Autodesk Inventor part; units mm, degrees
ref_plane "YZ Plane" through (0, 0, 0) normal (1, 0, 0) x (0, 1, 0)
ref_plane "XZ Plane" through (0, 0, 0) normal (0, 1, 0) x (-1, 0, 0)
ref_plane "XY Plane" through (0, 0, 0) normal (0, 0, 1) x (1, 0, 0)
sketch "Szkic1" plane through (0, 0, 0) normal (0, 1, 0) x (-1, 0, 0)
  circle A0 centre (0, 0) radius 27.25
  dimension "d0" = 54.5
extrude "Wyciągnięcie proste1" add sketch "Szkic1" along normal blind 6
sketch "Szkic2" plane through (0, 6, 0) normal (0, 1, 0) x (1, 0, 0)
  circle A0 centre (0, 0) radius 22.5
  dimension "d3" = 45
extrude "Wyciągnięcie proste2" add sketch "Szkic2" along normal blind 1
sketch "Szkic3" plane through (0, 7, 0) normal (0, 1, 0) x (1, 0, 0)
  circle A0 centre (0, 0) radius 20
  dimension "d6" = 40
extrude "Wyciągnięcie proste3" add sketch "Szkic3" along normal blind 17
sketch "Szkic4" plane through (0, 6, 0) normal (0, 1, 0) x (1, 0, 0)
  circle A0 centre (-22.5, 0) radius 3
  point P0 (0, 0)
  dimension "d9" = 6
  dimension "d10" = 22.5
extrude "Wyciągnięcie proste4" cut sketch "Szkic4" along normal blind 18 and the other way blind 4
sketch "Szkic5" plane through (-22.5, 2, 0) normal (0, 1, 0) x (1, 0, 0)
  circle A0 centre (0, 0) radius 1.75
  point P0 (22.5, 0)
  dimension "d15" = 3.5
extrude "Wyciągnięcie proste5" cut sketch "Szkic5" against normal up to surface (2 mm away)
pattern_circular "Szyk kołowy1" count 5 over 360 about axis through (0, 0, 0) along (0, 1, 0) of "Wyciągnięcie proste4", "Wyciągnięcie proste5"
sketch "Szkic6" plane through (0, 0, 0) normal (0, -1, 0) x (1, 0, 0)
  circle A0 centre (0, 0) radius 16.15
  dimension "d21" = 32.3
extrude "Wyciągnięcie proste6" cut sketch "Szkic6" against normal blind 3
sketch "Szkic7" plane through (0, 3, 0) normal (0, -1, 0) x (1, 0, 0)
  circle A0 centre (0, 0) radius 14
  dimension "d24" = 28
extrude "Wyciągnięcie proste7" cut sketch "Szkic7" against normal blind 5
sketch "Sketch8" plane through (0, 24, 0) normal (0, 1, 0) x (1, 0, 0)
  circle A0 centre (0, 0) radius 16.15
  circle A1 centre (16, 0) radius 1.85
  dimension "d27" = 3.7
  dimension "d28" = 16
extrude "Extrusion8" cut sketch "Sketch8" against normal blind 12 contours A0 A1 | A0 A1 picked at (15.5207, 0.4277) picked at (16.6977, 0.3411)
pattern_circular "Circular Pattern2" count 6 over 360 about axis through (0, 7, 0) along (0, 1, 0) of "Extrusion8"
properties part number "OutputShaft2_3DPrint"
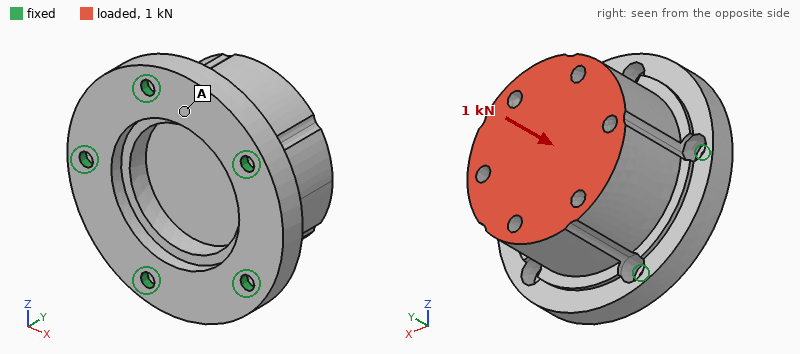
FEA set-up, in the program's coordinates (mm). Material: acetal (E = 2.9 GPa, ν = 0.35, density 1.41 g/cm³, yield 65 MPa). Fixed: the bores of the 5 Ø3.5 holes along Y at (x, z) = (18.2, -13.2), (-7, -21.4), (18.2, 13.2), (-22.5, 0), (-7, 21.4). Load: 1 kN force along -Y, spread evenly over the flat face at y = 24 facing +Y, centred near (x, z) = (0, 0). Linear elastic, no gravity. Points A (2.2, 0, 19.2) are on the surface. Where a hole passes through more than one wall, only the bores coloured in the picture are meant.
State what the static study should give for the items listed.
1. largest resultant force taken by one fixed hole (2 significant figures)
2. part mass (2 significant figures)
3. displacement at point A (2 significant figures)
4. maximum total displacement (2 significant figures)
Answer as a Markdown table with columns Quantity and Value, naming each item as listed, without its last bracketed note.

| Quantity | Value |
|---|---|
| largest resultant force taken by one fixed hole | 230 N |
| part mass | 42 g |
| displacement at point A | 31 µm |
| maximum total displacement | 41 µm |
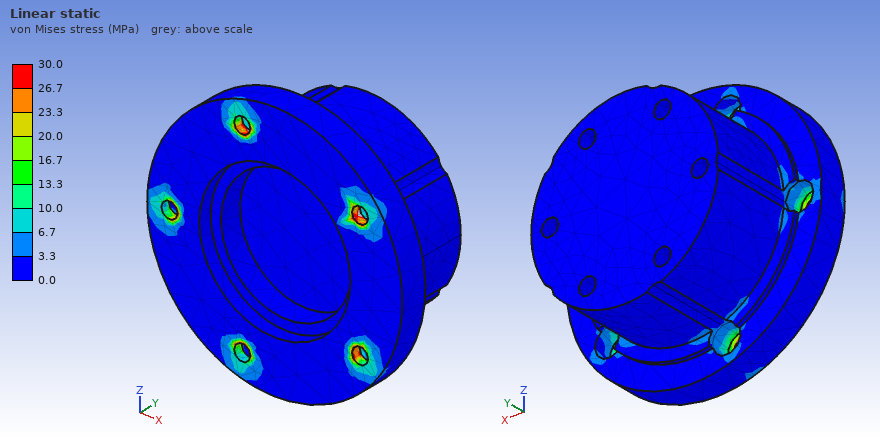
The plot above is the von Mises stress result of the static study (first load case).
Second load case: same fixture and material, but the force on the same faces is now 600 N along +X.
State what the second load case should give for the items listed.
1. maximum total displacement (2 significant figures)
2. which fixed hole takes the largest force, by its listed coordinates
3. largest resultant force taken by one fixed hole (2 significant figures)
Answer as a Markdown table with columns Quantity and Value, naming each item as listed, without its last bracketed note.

| Quantity | Value |
|---|---|
| maximum total displacement | 75 µm |
| which fixed hole takes the largest force, by its listed coordinates | (-22.5, 0) |
| largest resultant force taken by one fixed hole | 300 N |
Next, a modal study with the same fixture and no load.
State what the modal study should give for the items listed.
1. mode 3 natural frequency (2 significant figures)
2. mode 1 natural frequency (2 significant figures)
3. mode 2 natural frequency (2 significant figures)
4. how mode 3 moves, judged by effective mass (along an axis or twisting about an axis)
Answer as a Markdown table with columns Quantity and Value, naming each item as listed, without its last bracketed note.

| Quantity | Value |
|---|---|
| mode 3 natural frequency | 4400 Hz |
| mode 1 natural frequency | 3600 Hz |
| mode 2 natural frequency | 3600 Hz |
| how mode 3 moves, judged by effective mass | along Y |
